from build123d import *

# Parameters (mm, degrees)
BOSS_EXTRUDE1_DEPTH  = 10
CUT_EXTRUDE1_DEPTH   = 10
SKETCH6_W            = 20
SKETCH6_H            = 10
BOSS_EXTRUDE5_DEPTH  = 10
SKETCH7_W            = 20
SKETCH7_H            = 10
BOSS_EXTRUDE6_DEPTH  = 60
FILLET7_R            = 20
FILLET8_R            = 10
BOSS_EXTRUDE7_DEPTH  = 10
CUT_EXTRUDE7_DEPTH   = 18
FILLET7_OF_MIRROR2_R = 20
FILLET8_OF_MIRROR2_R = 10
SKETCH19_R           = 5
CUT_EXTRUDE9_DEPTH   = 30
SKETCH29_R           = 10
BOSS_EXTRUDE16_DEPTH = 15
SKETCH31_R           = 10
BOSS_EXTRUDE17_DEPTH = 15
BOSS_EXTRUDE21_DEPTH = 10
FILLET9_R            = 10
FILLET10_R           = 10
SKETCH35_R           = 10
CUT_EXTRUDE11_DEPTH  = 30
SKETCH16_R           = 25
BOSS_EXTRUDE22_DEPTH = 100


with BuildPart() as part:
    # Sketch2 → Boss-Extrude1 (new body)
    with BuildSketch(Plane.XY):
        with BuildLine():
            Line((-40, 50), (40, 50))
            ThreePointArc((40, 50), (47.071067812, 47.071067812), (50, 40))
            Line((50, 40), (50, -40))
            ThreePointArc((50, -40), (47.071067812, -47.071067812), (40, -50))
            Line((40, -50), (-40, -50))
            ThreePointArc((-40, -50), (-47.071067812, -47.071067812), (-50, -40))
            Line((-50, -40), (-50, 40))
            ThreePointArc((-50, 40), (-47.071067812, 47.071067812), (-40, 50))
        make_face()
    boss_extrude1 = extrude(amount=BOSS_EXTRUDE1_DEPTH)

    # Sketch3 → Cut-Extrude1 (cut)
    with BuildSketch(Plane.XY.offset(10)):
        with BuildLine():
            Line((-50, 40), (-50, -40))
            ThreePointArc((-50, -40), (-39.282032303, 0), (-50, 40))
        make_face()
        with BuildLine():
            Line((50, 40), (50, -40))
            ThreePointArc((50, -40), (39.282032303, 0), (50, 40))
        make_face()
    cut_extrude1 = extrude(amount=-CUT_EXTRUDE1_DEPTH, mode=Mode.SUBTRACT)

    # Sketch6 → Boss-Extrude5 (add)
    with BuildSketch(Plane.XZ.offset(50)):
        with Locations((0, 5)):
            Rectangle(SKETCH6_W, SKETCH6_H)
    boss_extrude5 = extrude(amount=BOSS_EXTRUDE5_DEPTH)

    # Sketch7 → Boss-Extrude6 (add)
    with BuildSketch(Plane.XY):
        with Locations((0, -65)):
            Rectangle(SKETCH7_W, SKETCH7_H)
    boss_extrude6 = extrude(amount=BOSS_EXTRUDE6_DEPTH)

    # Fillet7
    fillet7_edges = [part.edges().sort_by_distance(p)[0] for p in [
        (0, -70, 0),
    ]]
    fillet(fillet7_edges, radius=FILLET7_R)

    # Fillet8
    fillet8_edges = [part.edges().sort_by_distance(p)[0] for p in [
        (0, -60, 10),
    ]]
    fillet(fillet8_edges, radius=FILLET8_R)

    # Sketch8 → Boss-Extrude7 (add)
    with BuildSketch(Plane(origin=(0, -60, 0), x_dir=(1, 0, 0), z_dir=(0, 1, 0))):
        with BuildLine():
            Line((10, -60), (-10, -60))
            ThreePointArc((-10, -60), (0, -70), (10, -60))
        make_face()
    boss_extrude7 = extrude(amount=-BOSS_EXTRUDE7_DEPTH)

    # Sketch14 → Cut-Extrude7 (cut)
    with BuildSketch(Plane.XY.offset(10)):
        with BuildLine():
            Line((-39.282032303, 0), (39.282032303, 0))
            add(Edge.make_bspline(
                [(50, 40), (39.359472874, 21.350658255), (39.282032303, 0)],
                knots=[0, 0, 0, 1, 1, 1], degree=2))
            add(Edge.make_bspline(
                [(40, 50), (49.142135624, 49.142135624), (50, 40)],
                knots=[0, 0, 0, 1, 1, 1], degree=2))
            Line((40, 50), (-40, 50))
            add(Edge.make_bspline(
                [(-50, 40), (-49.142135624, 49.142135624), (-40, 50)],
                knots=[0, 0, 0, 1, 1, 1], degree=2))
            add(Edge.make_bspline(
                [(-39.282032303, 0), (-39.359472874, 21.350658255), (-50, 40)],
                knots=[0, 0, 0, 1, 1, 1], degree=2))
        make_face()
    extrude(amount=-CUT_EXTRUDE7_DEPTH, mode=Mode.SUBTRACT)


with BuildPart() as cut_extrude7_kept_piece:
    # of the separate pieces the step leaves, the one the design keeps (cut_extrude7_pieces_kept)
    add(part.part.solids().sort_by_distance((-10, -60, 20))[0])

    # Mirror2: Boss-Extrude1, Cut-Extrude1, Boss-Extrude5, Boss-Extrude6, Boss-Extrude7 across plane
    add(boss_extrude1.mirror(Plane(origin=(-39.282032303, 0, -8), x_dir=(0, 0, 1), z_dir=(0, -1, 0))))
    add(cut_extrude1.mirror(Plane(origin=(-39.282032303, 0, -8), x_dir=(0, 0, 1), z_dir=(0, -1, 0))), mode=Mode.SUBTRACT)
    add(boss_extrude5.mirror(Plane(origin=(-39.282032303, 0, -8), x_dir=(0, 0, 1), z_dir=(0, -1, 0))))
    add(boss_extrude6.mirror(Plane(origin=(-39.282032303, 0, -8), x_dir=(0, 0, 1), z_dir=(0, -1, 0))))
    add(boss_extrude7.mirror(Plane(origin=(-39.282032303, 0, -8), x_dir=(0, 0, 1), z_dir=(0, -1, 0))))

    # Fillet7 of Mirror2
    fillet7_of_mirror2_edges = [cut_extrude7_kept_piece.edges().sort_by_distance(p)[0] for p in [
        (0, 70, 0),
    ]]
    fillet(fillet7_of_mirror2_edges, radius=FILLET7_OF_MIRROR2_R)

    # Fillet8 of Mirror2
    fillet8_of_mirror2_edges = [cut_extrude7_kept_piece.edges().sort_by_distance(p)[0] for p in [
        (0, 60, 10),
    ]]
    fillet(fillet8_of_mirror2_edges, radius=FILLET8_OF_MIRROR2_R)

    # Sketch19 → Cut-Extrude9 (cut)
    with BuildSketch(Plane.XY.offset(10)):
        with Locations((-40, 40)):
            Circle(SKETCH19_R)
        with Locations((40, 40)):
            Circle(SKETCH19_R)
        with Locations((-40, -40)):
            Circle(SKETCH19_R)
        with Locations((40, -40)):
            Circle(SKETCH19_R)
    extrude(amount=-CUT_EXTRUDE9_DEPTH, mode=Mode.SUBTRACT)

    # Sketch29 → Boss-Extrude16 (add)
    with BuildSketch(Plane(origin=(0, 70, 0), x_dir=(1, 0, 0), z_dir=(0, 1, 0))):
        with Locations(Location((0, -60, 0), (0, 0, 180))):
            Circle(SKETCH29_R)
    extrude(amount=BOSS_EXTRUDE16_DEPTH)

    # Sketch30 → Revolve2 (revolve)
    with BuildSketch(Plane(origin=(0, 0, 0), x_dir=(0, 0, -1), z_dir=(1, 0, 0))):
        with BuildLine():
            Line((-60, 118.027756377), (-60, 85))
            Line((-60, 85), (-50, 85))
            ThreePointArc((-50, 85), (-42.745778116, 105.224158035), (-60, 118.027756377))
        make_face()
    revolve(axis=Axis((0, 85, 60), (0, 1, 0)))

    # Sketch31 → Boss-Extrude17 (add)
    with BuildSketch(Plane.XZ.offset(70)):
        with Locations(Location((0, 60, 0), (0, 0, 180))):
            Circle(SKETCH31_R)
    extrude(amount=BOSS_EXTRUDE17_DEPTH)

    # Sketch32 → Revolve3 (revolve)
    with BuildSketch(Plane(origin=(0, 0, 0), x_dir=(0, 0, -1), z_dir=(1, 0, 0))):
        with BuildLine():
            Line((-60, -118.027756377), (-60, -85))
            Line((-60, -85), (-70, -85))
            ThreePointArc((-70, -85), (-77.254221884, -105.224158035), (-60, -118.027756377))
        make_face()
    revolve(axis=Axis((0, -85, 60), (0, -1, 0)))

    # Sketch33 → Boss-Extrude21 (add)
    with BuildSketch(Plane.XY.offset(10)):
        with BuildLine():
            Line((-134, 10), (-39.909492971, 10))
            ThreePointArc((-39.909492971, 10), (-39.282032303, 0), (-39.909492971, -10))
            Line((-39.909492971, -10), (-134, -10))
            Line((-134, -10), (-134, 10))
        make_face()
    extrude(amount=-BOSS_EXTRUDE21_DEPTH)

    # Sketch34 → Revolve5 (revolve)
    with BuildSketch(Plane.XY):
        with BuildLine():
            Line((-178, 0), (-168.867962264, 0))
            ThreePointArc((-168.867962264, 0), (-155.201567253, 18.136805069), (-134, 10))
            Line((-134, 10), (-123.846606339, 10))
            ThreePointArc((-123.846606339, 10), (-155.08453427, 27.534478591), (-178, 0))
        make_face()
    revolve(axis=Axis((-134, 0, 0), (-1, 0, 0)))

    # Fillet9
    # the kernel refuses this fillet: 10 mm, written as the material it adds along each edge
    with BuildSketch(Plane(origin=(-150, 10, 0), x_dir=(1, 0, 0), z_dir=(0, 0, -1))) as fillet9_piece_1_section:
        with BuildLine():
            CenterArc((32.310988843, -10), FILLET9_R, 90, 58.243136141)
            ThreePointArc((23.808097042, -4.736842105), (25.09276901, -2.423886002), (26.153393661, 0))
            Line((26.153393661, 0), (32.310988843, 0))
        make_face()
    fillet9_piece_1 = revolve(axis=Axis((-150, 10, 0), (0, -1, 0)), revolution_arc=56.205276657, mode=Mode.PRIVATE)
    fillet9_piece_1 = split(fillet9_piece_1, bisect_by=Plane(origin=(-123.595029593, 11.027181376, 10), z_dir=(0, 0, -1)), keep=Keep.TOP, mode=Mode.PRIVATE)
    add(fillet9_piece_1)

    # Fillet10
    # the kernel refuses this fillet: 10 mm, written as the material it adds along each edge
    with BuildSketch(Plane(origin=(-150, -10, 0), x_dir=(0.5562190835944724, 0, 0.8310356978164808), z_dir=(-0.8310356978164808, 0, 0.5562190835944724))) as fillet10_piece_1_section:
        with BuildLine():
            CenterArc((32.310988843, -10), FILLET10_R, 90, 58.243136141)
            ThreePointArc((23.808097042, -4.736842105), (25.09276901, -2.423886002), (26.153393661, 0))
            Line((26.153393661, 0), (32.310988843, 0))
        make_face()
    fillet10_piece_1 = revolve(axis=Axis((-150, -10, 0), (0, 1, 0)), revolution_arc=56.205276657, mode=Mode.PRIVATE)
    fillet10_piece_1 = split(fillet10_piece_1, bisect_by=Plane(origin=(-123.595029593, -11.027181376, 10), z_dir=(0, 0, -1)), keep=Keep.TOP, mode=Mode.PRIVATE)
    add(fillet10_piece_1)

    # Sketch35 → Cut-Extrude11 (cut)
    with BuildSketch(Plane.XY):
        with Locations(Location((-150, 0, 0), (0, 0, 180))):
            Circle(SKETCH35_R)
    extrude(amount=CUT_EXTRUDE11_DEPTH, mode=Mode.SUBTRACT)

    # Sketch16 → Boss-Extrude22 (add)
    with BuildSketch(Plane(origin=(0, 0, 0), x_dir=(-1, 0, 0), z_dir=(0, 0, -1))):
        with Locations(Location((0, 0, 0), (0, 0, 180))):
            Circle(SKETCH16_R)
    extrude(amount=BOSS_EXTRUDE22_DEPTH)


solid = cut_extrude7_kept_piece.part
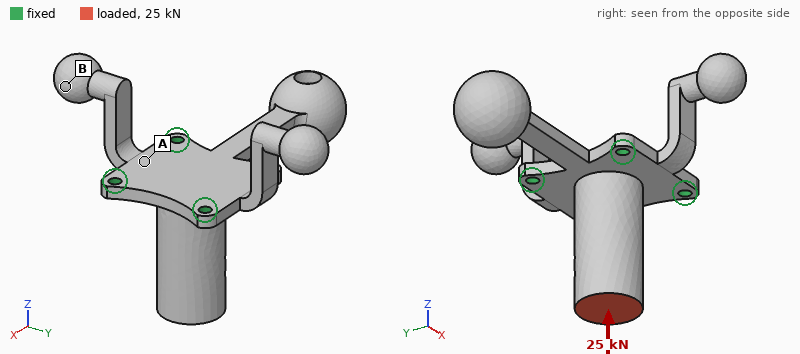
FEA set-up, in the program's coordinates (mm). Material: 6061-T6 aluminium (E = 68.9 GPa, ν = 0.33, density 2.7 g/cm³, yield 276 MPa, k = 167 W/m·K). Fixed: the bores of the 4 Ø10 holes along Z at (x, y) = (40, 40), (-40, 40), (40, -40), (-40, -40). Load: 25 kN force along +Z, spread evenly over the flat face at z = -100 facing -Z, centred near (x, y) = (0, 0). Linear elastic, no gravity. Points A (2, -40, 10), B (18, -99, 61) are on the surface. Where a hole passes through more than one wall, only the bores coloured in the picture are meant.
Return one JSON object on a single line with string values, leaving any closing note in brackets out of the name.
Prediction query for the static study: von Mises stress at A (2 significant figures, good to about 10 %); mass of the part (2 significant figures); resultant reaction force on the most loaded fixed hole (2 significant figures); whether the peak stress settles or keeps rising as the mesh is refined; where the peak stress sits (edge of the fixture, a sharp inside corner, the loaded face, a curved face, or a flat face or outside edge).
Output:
{"von Mises stress at A": "55 MPa", "mass of the part": "1.2 kg", "resultant reaction force on the most loaded fixed hole": "6.5 kN", "whether the peak stress settles or keeps rising as the mesh is refined": "keeps rising", "where the peak stress sits": "edge of the fixture"}
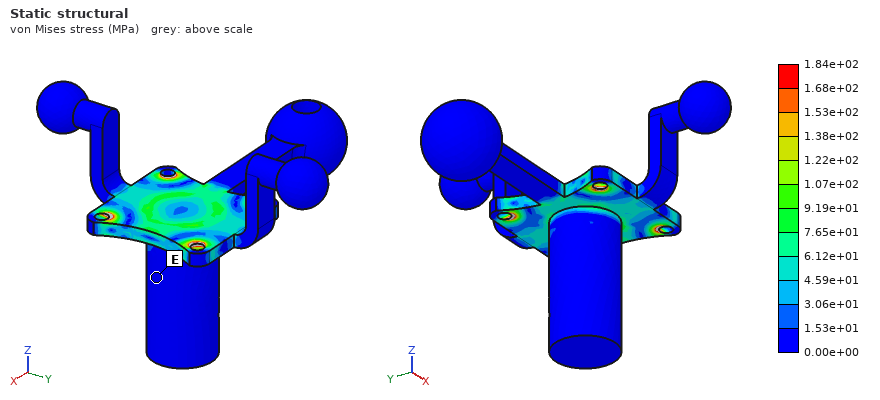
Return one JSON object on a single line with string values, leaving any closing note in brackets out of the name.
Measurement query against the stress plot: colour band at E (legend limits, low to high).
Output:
{"colour band at E": "0.00e+00 to 1.53e+01 MPa"}
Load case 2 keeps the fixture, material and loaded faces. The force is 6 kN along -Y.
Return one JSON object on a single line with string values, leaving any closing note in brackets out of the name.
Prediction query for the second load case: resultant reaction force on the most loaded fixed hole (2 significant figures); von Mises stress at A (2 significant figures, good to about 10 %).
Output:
{"resultant reaction force on the most loaded fixed hole": "4.9 kN", "von Mises stress at A": "56 MPa"}
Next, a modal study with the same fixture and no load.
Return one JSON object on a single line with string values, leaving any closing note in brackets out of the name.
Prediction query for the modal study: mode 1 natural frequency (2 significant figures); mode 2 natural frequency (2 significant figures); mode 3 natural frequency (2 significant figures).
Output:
{"mode 1 natural frequency": "170 Hz", "mode 2 natural frequency": "340 Hz", "mode 3 natural frequency": "380 Hz"}
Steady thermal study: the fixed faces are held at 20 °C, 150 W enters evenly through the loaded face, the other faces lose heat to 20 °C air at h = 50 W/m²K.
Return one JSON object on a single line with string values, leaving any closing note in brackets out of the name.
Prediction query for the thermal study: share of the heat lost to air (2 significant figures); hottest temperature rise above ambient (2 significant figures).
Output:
{"share of the heat lost to air": "30 %", "hottest temperature rise above ambient": "58 K"}
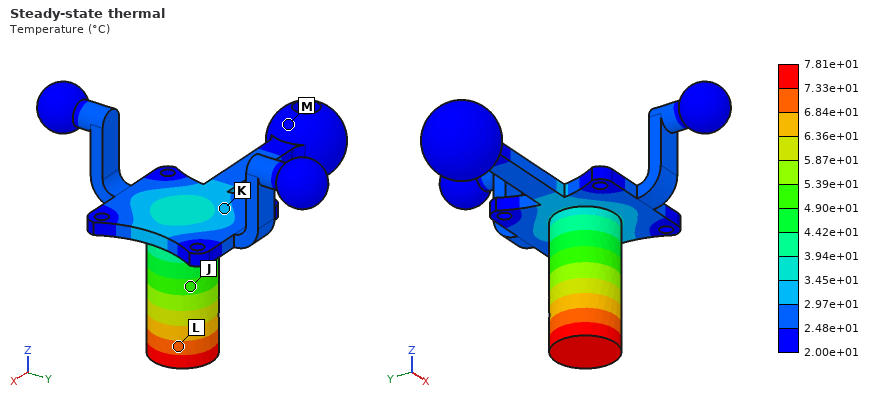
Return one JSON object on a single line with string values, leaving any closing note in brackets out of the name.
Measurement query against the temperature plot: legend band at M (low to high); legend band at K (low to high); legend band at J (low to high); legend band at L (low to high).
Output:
{"legend band at M": "2.00e+01 to 2.48e+01 °C", "legend band at K": "2.97e+01 to 3.45e+01 °C", "legend band at J": "4.90e+01 to 5.39e+01 °C", "legend band at L": "6.84e+01 to 7.33e+01 °C"}
